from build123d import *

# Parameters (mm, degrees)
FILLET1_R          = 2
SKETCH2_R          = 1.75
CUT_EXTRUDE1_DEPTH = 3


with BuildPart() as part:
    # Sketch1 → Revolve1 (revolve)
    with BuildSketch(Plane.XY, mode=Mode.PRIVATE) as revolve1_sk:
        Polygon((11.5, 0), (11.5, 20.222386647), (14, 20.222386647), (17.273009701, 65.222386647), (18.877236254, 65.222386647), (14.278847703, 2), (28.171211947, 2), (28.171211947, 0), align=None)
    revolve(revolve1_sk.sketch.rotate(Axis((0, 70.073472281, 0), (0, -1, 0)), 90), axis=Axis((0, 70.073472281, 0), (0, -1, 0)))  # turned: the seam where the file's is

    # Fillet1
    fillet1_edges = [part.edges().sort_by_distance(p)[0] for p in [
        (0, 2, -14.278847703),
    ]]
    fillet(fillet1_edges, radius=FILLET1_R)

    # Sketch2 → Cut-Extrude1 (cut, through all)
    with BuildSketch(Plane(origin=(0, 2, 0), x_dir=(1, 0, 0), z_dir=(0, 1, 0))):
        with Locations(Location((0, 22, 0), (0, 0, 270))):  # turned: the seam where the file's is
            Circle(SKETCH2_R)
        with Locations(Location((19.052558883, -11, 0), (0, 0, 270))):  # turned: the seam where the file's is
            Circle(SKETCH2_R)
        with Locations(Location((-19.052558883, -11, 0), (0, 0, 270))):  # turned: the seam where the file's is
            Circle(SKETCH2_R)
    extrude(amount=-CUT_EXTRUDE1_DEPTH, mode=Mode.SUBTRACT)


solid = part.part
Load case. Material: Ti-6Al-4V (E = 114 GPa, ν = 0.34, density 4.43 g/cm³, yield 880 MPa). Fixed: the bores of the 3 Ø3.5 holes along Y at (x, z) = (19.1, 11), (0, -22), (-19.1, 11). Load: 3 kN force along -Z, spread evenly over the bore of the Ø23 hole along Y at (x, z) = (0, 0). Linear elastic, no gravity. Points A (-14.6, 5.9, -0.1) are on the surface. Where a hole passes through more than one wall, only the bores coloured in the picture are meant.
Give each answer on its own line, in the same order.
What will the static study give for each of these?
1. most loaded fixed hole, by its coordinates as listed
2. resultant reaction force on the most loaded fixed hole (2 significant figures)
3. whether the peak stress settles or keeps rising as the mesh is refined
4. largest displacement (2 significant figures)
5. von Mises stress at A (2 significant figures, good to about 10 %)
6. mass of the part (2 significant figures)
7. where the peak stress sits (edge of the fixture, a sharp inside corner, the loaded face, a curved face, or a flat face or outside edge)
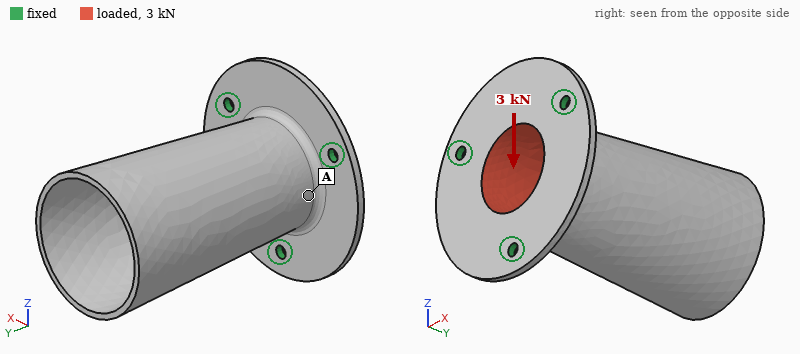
(0, -22)
1.4 kN
keeps rising
0.16 mm
24 MPa
75 g
edge of the fixture
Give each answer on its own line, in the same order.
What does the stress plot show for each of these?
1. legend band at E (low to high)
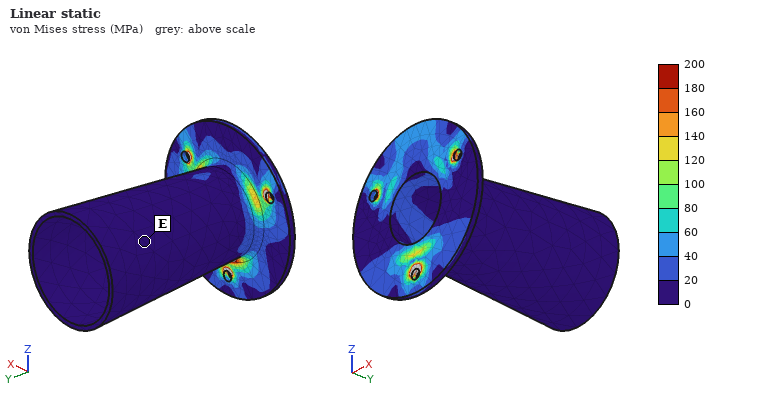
0 to 20 MPa
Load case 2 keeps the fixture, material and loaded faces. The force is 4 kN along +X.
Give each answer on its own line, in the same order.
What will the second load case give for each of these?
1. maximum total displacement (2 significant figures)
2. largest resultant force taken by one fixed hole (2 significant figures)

0.20 mm
1.7 kN
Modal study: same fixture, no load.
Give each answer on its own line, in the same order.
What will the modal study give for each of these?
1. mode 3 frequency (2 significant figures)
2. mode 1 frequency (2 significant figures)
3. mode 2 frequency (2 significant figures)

4200 Hz
1900 Hz
1900 Hz
